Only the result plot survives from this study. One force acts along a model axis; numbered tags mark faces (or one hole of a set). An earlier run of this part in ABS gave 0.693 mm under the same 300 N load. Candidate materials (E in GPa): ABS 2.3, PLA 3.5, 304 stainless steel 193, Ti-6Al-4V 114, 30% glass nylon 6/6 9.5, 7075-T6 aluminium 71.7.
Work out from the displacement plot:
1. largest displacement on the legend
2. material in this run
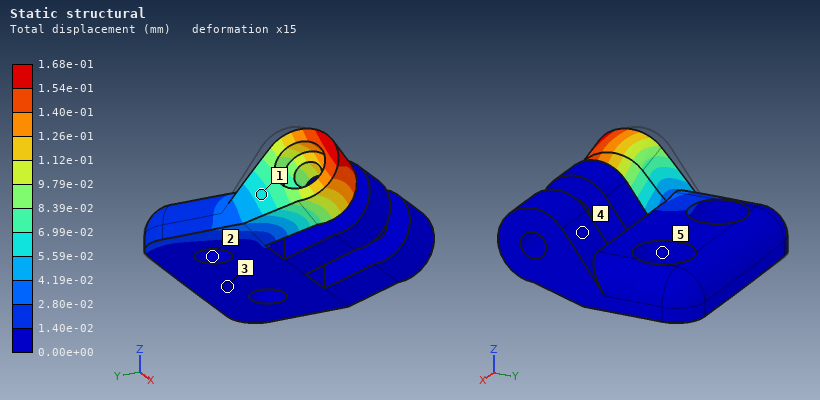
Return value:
1.68e-01 mm
30% glass nylon 6/6
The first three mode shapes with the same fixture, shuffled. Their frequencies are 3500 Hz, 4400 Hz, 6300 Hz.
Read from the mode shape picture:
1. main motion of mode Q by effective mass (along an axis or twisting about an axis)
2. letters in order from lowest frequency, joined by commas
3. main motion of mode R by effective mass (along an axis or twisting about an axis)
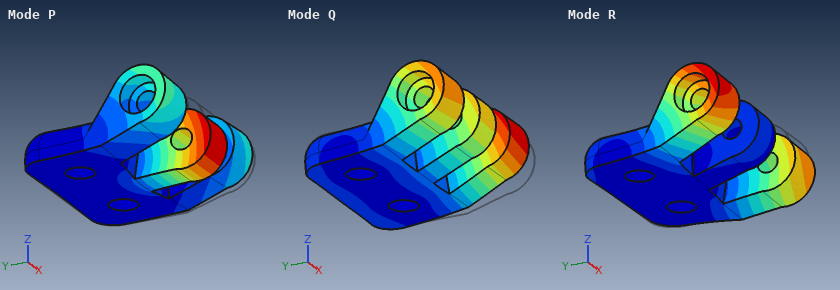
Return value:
along Z
Q, R, P
twisting about Y
